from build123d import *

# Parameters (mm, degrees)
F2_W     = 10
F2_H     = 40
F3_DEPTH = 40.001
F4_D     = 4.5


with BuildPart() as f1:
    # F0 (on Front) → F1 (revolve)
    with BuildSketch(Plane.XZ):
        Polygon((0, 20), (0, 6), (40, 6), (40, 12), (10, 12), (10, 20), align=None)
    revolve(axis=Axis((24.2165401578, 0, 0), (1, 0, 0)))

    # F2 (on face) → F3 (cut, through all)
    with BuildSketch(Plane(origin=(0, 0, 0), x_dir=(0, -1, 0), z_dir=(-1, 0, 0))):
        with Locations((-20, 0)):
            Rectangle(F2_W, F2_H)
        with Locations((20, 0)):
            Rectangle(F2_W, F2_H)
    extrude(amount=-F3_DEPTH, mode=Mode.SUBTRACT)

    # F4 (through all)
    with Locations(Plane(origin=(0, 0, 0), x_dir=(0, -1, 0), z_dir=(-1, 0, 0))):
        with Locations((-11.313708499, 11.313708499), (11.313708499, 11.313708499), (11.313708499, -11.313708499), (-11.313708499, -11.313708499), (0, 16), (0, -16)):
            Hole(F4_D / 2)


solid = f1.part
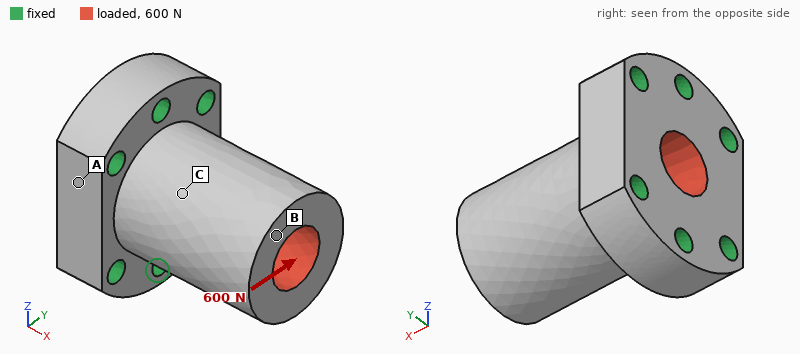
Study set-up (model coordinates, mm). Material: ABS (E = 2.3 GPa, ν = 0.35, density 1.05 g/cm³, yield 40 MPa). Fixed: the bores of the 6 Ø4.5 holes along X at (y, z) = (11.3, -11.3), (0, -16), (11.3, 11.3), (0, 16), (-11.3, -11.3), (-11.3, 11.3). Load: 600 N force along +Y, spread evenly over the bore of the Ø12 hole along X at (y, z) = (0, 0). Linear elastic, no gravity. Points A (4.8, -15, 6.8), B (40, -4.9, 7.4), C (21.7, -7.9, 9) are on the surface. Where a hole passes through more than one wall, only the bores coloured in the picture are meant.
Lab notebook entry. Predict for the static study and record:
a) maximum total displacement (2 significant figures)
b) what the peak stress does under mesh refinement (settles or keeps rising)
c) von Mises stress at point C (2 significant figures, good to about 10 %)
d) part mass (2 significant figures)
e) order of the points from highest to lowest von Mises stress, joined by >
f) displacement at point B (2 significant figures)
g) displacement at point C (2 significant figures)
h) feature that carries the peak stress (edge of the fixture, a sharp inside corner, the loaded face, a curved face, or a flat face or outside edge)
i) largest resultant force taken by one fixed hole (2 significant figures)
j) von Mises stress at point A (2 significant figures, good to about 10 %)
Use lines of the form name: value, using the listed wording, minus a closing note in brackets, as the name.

maximum total displacement: 0.14 mm
what the peak stress does under mesh refinement: keeps rising
von Mises stress at point C: 1.9 MPa
part mass: 20 g
order of the points from highest to lowest von Mises stress, joined by >: A > C > B
displacement at point B: 0.13 mm
displacement at point C: 0.063 mm
feature that carries the peak stress: edge of the fixture
largest resultant force taken by one fixed hole: 240 N
von Mises stress at point A: 3.8 MPa
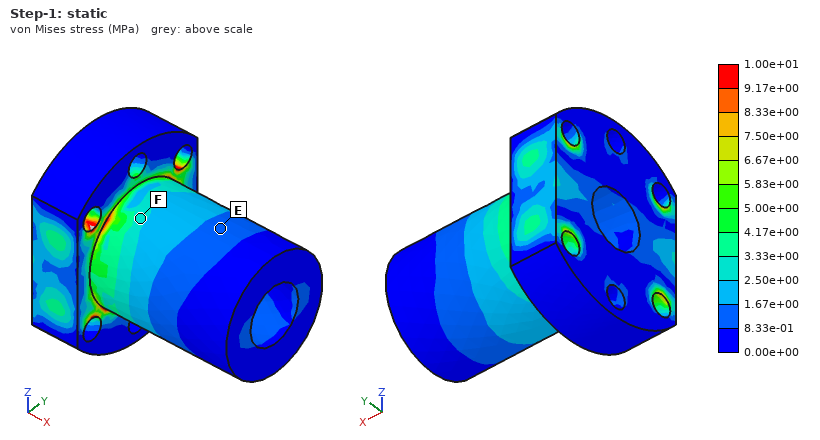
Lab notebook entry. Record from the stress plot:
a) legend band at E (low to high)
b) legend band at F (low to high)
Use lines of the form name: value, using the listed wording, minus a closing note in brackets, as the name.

legend band at E: 8.33e-01 to 1.67e+00 MPa
legend band at F: 2.50e+00 to 3.33e+00 MPa
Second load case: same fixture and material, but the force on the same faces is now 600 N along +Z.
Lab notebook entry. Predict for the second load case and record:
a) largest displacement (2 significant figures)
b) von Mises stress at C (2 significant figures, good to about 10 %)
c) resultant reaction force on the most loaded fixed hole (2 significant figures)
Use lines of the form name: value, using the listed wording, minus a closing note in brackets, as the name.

largest displacement: 0.12 mm
von Mises stress at C: 1.9 MPa
resultant reaction force on the most loaded fixed hole: 200 N
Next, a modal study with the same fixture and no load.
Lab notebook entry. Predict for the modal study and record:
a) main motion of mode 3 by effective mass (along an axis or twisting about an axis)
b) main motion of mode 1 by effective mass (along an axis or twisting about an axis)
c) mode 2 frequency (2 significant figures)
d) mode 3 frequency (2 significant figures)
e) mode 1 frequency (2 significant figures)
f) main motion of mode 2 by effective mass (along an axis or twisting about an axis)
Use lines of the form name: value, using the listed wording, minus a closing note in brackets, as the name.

main motion of mode 3 by effective mass: twisting about X
main motion of mode 1 by effective mass: along Y
mode 2 frequency: 3600 Hz
mode 3 frequency: 6800 Hz
mode 1 frequency: 3300 Hz
main motion of mode 2 by effective mass: along Z
